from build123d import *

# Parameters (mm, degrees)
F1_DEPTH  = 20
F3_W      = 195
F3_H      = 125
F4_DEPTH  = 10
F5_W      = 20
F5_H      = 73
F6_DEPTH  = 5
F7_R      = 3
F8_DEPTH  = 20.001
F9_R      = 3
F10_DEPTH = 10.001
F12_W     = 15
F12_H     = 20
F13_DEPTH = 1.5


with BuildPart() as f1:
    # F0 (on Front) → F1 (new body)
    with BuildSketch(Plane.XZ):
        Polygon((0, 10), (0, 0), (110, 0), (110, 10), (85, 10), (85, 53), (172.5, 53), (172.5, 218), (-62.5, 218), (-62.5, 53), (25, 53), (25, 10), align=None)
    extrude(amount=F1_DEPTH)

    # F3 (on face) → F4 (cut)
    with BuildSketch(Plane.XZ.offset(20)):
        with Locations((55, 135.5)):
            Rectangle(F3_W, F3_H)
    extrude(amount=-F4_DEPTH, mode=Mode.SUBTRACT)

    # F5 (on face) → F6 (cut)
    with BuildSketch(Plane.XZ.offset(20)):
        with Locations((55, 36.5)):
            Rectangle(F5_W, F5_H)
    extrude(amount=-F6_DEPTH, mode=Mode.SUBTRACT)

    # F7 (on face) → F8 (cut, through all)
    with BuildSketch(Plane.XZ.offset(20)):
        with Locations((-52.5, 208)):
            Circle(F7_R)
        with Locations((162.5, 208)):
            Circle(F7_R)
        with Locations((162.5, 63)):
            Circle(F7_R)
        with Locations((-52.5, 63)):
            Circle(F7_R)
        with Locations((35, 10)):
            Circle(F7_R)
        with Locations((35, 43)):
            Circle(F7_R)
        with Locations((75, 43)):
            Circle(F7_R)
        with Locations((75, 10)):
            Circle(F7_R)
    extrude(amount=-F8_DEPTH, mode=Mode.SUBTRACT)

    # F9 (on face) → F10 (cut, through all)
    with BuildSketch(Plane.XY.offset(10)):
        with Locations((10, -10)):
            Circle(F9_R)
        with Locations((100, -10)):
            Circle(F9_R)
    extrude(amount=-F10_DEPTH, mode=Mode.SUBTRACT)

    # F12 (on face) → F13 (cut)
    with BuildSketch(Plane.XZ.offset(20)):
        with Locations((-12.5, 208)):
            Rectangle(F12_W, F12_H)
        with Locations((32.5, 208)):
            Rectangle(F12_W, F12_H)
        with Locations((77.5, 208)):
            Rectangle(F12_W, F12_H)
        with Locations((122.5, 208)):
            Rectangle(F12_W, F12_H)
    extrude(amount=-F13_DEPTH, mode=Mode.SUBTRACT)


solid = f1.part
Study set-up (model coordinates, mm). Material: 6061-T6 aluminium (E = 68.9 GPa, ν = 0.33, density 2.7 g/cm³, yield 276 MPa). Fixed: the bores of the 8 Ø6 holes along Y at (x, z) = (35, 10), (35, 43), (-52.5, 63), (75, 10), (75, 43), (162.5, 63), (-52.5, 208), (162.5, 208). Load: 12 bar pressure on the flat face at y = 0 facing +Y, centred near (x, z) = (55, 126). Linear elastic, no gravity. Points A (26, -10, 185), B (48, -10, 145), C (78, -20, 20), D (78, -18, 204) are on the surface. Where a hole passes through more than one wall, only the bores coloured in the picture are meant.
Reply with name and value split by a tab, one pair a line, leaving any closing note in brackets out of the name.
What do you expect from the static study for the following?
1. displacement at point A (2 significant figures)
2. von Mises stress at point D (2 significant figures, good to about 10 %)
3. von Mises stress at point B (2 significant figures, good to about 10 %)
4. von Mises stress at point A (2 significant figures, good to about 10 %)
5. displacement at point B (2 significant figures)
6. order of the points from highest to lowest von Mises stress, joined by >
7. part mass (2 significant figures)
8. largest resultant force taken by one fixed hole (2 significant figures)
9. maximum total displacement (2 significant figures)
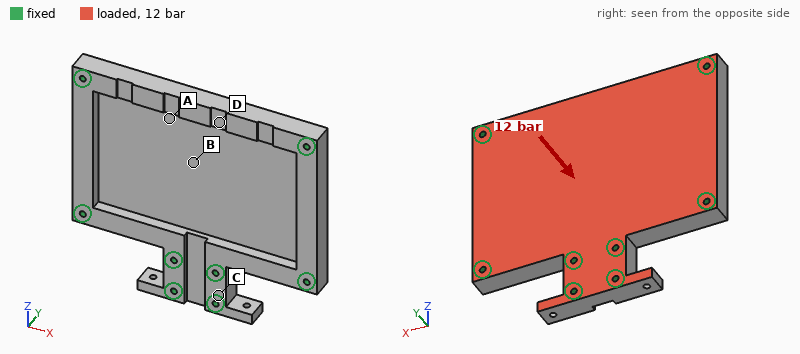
displacement at point A	0.41 mm
von Mises stress at point D	89 MPa
von Mises stress at point B	58 MPa
von Mises stress at point A	31 MPa
displacement at point B	0.49 mm
order of the points from highest to lowest von Mises stress, joined by >	D > B > A > C
part mass	1.6 kg
largest resultant force taken by one fixed hole	14 kN
maximum total displacement	0.51 mm
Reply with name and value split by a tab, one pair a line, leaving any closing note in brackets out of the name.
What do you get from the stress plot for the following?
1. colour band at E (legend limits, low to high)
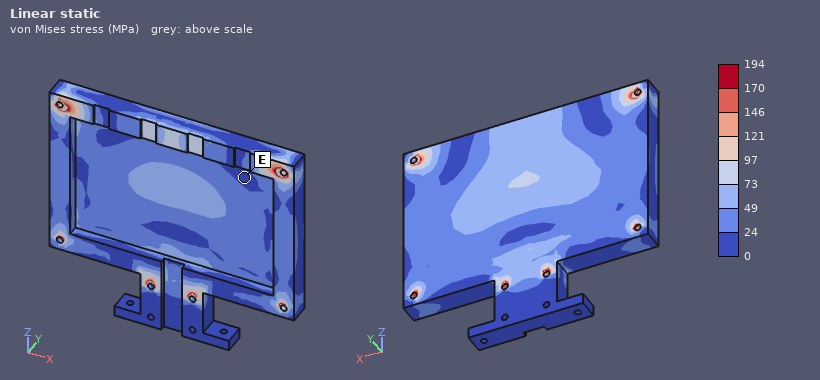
colour band at E	0 to 24 MPa
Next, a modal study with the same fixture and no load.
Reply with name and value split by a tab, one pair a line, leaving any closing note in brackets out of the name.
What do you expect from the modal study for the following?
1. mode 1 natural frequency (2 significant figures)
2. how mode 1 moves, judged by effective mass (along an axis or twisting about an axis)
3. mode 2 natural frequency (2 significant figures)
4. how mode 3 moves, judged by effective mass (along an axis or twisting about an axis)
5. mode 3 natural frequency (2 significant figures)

mode 1 natural frequency	1700 Hz
how mode 1 moves, judged by effective mass	along Y
mode 2 natural frequency	2800 Hz
how mode 3 moves, judged by effective mass	twisting about Z
mode 3 natural frequency	3200 Hz
